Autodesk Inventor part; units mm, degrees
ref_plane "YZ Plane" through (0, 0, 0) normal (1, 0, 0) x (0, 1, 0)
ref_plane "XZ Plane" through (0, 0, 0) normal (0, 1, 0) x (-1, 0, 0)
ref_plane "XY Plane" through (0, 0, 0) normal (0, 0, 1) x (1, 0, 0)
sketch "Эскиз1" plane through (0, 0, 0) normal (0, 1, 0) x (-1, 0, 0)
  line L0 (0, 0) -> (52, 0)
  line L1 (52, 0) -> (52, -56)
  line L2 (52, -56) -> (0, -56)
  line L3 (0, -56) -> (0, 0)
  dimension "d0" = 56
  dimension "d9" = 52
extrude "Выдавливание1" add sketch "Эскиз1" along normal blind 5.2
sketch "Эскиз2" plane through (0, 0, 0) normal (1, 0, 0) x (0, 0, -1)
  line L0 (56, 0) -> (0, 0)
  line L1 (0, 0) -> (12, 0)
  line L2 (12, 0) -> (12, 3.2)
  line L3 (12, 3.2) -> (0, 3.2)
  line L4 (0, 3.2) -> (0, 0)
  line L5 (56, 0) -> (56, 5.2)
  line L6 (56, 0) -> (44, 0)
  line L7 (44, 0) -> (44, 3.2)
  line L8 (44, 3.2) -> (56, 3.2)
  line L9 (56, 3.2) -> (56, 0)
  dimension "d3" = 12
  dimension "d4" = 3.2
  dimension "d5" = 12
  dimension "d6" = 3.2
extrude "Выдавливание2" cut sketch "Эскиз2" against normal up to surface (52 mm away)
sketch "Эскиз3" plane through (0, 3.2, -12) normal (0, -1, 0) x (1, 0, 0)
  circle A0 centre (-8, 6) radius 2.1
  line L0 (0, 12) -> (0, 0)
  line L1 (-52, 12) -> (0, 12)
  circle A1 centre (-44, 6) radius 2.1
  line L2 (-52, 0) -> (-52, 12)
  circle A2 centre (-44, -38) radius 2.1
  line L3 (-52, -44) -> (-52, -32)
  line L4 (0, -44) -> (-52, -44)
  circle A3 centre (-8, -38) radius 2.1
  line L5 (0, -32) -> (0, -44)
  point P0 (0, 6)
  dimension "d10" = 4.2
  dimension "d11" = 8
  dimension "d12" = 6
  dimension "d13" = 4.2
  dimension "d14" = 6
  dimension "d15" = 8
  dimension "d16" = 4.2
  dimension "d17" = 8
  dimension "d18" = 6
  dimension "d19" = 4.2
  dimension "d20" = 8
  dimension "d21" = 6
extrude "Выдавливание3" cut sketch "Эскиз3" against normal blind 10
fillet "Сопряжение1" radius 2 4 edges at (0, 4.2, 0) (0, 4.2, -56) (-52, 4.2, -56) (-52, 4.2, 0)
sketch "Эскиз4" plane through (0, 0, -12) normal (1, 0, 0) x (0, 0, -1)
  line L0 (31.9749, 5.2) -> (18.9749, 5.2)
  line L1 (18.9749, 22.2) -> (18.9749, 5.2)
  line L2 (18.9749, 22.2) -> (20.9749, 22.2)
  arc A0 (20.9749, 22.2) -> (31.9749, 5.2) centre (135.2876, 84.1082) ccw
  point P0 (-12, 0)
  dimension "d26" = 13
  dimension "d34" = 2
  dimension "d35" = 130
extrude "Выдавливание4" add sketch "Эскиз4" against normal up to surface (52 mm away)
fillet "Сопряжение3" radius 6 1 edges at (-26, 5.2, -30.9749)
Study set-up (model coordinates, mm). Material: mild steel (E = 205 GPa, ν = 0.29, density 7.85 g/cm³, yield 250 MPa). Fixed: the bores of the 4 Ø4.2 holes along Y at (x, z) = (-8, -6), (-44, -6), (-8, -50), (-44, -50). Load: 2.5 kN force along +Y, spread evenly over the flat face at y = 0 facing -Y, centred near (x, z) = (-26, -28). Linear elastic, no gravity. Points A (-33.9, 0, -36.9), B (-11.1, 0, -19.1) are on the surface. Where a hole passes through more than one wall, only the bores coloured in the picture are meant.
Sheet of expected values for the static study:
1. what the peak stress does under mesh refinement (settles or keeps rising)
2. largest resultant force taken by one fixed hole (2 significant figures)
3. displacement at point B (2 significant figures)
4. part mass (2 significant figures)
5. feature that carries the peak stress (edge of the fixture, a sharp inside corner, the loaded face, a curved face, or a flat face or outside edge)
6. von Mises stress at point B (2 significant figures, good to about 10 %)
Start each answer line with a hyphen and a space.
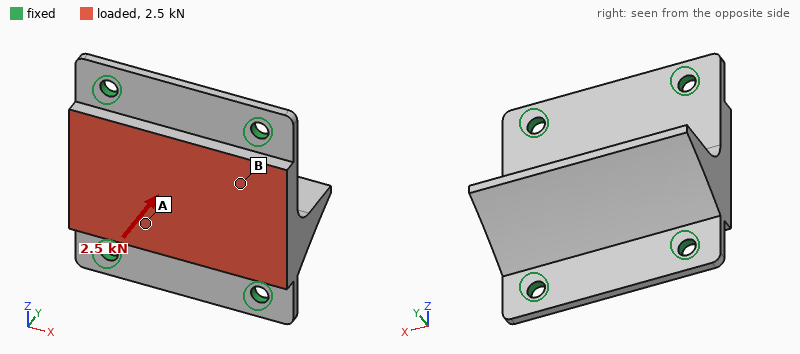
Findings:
- keeps rising
- 810 N
- 14 µm
- 140 g
- edge of the fixture
- 41 MPa
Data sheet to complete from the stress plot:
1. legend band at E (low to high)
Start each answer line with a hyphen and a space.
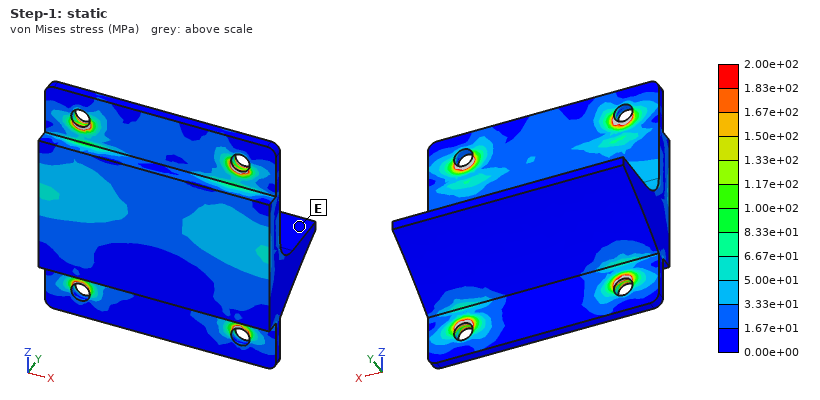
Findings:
- 0.00e+00 to 1.67e+01 MPa
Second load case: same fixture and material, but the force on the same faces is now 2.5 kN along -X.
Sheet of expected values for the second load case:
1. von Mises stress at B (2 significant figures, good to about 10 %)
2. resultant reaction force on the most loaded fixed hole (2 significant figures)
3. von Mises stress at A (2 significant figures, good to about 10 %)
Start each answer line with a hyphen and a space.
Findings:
- 11 MPa
- 690 N
- 9.6 MPa
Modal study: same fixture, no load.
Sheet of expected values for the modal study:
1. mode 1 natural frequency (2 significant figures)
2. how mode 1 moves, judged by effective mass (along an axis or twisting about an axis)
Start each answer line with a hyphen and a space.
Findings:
- 6000 Hz
- along Y
